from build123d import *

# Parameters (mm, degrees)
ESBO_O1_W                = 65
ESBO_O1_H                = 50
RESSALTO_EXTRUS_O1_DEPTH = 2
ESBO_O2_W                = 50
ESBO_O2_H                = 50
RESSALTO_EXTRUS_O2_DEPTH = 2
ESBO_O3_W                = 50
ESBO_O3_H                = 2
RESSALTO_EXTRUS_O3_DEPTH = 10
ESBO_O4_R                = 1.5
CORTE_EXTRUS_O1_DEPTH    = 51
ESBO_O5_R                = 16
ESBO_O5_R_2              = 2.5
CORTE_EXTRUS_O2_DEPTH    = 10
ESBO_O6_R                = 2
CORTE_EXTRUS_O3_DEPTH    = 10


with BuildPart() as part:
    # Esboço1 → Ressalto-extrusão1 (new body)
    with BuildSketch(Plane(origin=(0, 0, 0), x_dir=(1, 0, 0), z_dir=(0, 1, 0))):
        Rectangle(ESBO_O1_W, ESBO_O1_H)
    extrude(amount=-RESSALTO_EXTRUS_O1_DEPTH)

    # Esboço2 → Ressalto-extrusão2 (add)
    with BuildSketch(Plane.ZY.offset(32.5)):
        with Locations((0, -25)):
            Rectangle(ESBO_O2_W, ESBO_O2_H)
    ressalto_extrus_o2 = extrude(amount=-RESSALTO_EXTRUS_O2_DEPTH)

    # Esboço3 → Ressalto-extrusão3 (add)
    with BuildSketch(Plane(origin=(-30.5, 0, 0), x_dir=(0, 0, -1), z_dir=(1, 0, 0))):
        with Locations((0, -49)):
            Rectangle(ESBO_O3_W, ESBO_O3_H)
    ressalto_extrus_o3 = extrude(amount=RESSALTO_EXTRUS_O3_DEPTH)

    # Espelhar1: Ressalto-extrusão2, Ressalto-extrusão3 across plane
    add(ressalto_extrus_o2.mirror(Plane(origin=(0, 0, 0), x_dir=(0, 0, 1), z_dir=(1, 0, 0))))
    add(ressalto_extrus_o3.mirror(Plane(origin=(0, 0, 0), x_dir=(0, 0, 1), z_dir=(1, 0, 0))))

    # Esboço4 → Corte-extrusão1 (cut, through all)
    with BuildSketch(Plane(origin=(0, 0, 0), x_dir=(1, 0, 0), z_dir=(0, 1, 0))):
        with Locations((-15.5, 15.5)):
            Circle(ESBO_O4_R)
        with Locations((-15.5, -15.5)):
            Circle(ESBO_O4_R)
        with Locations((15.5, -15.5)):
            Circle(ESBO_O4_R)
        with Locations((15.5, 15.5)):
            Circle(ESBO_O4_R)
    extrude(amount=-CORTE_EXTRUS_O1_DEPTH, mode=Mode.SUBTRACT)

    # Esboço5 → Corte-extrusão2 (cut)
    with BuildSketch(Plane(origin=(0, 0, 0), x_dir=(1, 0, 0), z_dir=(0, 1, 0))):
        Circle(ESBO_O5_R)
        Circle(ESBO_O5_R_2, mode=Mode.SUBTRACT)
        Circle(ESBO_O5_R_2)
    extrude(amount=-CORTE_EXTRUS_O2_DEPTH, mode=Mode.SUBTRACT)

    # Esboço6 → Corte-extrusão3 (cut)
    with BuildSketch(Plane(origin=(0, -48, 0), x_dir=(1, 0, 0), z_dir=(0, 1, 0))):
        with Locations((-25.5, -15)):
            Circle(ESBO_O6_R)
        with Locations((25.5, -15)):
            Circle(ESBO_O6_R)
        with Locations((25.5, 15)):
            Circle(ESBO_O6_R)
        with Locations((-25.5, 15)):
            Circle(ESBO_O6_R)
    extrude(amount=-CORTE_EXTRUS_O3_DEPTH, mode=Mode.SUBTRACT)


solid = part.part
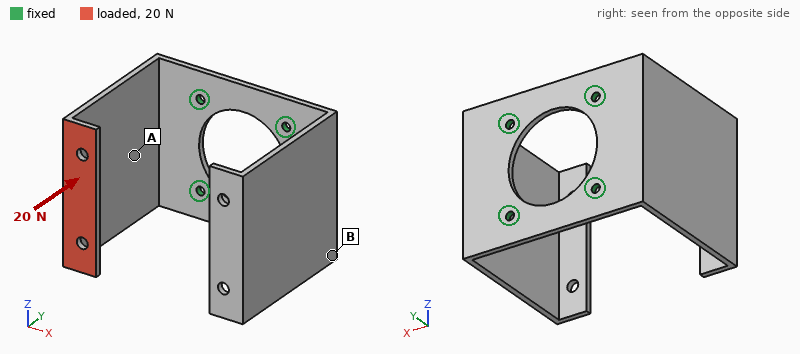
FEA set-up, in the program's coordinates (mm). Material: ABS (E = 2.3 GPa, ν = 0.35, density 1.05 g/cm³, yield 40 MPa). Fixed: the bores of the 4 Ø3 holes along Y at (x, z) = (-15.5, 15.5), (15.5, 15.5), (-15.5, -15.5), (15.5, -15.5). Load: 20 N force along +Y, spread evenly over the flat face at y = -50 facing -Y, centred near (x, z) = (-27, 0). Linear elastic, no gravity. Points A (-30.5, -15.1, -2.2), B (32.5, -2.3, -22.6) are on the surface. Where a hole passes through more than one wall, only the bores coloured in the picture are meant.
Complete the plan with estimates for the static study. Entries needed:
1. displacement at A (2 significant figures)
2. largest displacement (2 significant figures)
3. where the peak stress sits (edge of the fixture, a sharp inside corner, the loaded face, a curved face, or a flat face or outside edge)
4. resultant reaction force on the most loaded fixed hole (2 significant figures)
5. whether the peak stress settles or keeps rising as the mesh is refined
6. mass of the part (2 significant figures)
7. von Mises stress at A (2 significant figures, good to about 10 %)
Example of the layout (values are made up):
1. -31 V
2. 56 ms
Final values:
1. 0.28 mm
2. 0.93 mm
3. edge of the fixture
4. 10 N
5. keeps rising
6. 17 g
7. 2.8 MPa
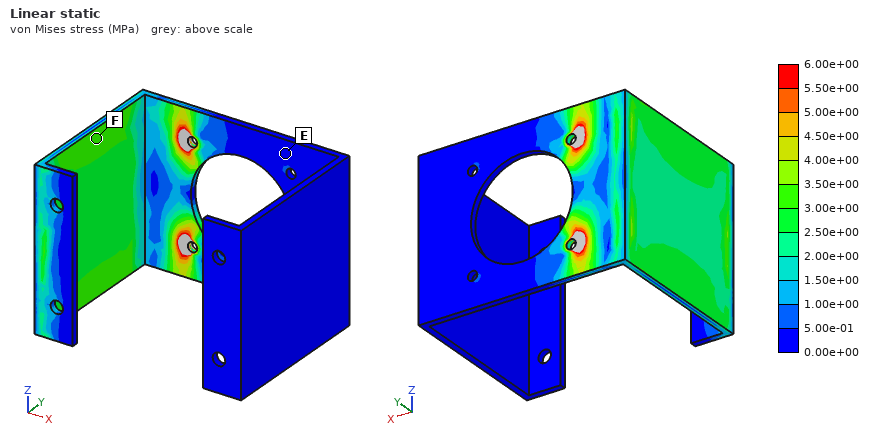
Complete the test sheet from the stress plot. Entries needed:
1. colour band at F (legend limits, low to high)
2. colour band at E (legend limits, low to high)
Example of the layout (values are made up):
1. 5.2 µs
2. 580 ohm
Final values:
1. 3.00e+00 to 3.50e+00 MPa
2. 0.00e+00 to 5.00e-01 MPa
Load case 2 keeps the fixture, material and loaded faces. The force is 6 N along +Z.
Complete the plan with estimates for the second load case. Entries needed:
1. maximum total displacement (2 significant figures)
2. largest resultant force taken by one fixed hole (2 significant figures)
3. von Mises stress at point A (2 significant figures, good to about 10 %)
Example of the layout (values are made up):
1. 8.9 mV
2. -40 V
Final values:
1. 0.94 mm
2. 9.3 N
3. 1.4 MPa
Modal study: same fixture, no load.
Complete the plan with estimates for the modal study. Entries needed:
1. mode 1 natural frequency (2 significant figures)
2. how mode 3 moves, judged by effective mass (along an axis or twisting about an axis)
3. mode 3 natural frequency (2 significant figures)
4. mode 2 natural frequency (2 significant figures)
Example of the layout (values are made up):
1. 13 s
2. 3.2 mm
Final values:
1. 100 Hz
2. along Z
3. 260 Hz
4. 100 Hz
